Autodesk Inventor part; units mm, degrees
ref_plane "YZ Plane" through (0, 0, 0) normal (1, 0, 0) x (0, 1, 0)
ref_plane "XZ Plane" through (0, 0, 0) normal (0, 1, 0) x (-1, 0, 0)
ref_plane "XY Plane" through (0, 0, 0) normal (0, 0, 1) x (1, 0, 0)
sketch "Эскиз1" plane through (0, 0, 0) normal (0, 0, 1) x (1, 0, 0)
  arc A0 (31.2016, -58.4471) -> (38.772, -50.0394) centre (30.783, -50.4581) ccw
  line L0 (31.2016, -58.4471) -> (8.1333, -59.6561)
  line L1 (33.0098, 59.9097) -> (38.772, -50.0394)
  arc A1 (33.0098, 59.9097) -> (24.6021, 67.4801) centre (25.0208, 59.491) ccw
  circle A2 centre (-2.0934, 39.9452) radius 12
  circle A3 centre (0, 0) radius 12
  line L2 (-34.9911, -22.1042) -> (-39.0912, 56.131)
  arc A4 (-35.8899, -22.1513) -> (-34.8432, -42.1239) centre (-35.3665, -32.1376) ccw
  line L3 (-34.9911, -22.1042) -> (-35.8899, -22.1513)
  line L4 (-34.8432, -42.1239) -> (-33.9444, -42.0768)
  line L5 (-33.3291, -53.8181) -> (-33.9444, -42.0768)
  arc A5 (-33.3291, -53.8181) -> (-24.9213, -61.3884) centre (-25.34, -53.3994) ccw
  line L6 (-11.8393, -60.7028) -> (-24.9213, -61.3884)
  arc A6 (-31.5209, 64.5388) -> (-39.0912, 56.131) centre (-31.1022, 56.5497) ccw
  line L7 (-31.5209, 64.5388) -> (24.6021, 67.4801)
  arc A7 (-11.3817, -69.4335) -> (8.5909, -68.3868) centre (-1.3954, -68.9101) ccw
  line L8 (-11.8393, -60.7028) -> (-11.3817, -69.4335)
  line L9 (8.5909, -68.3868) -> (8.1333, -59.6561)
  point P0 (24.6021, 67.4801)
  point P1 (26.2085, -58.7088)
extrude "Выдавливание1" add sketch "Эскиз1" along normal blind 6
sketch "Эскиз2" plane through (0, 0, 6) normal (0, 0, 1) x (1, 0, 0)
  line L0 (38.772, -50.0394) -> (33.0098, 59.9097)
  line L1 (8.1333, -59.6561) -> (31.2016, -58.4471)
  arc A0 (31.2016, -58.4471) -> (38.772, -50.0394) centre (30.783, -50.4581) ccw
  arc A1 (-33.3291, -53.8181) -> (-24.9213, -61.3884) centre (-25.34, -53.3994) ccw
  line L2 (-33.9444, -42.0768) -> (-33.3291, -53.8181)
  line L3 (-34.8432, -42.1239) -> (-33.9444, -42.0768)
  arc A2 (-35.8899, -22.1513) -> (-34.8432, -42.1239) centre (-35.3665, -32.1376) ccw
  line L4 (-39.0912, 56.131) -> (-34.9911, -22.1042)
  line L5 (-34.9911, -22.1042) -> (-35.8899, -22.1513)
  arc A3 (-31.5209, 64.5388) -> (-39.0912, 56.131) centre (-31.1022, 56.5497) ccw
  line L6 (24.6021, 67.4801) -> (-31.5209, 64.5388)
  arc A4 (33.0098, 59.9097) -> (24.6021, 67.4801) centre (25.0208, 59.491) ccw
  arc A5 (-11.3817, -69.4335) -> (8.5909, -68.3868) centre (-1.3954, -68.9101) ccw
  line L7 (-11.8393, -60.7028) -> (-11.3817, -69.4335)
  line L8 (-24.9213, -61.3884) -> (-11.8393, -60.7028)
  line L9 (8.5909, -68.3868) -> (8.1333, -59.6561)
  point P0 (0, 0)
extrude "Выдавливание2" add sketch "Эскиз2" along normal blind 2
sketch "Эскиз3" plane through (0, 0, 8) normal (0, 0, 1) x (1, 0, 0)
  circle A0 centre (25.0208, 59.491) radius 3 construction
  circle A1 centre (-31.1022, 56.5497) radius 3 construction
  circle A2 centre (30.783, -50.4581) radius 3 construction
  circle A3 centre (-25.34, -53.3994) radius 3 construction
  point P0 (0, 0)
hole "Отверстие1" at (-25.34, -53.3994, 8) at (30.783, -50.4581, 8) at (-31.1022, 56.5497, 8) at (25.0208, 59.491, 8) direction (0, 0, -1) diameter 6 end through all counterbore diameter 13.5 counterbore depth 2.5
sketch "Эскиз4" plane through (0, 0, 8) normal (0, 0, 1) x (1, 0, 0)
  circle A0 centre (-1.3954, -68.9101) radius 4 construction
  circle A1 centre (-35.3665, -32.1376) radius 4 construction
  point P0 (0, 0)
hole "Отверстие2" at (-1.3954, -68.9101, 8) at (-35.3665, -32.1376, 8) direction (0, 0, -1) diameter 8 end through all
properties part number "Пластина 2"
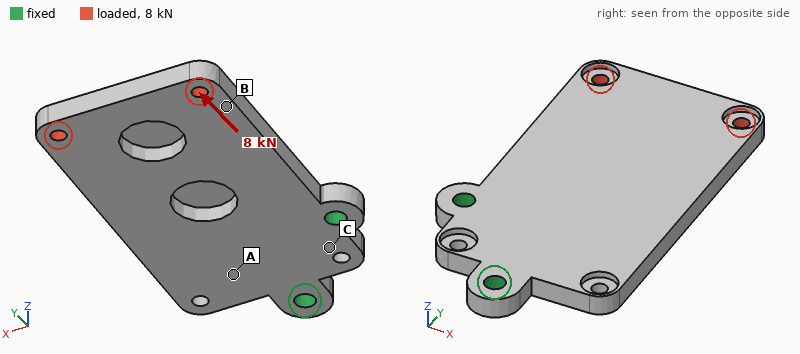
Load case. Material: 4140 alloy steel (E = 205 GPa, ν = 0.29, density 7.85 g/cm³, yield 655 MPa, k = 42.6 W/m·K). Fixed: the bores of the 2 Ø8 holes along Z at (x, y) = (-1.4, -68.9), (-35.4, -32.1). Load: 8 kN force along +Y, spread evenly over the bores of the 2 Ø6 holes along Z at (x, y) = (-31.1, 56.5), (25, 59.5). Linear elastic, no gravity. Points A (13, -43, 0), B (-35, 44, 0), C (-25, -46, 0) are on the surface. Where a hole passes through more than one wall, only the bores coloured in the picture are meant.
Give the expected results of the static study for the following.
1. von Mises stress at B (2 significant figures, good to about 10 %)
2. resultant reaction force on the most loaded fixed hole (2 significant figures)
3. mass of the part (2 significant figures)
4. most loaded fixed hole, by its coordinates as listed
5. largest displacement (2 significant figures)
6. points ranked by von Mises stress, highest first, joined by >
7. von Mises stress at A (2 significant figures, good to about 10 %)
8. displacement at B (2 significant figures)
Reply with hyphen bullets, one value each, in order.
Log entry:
- 48 MPa
- 5.8 kN
- 540 g
- (-1.4, -68.9)
- 0.13 mm
- B > A > C
- 30 MPa
- 0.073 mm
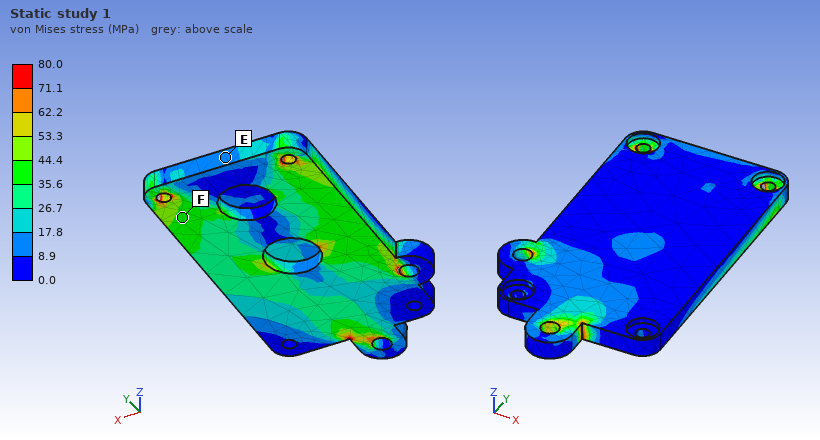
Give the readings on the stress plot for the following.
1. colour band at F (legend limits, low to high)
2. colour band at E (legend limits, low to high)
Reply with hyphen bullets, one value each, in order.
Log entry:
- 35.6 to 44.4 MPa
- 8.9 to 17.8 MPa
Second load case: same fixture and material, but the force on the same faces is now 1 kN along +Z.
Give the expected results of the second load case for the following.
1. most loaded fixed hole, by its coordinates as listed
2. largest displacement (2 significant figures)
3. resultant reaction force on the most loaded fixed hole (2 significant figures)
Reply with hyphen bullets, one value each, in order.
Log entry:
- (-35.4, -32.1)
- 0.82 mm
- 1.8 kN
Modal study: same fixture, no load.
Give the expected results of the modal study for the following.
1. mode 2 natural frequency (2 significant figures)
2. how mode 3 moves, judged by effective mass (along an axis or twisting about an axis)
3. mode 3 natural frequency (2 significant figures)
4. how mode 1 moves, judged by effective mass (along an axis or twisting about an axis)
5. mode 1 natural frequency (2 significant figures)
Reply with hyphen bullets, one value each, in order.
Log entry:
- 1400 Hz
- along Z
- 2700 Hz
- along Z
- 520 Hz
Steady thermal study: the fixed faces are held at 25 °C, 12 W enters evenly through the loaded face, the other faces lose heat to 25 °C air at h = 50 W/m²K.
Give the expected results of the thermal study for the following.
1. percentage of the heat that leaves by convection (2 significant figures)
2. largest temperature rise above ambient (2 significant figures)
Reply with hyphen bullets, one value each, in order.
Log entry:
- 83 %
- 31 K
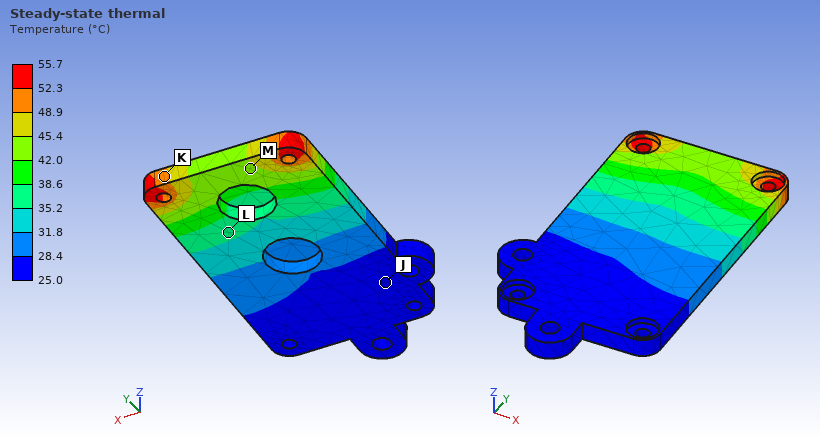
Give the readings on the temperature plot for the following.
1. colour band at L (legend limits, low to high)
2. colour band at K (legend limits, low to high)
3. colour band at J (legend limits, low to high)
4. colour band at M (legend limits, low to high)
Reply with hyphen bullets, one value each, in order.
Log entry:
- 35.2 to 38.6 °C
- 48.9 to 52.3 °C
- 25.0 to 28.4 °C
- 42.0 to 45.4 °C
